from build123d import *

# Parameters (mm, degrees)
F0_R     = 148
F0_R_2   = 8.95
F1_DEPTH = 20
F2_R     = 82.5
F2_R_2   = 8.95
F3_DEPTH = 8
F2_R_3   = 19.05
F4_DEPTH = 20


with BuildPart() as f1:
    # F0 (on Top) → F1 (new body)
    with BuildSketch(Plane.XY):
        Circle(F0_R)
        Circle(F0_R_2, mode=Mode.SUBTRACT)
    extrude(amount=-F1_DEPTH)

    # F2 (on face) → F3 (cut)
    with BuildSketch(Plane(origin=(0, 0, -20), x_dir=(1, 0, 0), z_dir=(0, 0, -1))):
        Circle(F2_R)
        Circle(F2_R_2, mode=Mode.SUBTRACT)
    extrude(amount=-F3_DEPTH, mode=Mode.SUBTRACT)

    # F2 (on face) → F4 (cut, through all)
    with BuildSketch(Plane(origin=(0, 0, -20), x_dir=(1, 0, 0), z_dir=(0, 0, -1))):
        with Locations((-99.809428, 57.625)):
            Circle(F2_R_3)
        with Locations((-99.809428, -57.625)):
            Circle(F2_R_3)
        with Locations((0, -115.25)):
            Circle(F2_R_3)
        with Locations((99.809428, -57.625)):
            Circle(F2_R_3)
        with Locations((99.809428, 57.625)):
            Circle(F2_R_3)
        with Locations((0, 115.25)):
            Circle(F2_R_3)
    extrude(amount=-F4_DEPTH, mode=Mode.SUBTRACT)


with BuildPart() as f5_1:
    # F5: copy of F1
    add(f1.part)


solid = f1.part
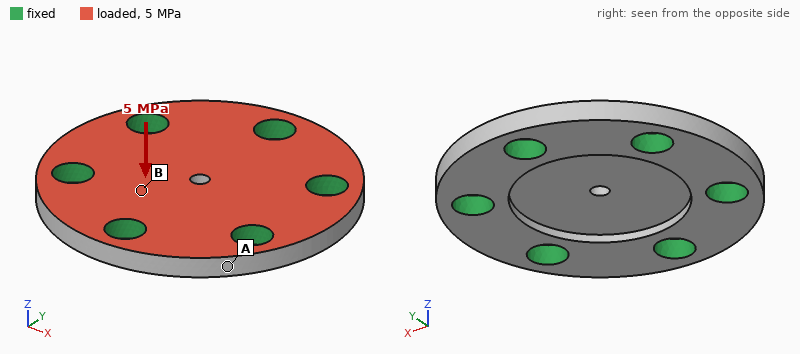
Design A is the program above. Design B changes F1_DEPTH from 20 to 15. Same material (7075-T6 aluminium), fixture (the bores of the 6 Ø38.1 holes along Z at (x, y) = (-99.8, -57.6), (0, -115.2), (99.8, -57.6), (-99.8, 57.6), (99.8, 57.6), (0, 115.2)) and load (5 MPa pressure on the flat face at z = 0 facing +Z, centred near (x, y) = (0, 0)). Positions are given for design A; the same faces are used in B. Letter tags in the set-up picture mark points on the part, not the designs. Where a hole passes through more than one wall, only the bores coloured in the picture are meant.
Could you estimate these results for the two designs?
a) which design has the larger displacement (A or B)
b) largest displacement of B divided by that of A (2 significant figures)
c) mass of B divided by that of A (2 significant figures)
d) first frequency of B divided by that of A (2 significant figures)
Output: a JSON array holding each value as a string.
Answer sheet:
["B", "1.2", "0.81", "0.91"]
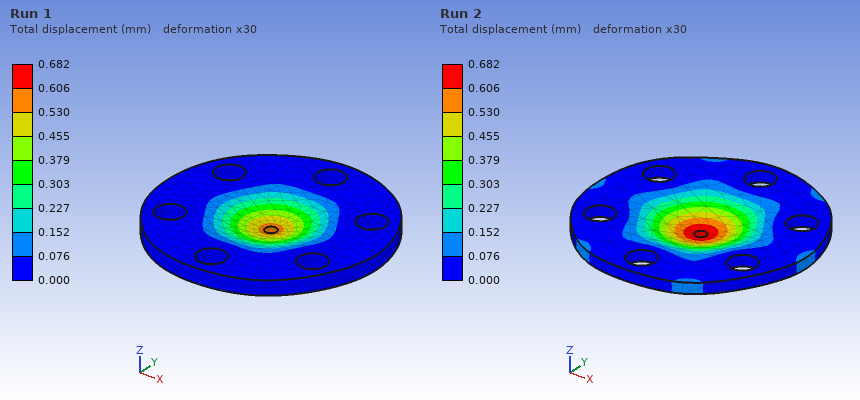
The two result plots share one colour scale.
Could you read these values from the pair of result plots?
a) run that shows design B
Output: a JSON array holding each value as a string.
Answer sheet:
["Run 2"]
